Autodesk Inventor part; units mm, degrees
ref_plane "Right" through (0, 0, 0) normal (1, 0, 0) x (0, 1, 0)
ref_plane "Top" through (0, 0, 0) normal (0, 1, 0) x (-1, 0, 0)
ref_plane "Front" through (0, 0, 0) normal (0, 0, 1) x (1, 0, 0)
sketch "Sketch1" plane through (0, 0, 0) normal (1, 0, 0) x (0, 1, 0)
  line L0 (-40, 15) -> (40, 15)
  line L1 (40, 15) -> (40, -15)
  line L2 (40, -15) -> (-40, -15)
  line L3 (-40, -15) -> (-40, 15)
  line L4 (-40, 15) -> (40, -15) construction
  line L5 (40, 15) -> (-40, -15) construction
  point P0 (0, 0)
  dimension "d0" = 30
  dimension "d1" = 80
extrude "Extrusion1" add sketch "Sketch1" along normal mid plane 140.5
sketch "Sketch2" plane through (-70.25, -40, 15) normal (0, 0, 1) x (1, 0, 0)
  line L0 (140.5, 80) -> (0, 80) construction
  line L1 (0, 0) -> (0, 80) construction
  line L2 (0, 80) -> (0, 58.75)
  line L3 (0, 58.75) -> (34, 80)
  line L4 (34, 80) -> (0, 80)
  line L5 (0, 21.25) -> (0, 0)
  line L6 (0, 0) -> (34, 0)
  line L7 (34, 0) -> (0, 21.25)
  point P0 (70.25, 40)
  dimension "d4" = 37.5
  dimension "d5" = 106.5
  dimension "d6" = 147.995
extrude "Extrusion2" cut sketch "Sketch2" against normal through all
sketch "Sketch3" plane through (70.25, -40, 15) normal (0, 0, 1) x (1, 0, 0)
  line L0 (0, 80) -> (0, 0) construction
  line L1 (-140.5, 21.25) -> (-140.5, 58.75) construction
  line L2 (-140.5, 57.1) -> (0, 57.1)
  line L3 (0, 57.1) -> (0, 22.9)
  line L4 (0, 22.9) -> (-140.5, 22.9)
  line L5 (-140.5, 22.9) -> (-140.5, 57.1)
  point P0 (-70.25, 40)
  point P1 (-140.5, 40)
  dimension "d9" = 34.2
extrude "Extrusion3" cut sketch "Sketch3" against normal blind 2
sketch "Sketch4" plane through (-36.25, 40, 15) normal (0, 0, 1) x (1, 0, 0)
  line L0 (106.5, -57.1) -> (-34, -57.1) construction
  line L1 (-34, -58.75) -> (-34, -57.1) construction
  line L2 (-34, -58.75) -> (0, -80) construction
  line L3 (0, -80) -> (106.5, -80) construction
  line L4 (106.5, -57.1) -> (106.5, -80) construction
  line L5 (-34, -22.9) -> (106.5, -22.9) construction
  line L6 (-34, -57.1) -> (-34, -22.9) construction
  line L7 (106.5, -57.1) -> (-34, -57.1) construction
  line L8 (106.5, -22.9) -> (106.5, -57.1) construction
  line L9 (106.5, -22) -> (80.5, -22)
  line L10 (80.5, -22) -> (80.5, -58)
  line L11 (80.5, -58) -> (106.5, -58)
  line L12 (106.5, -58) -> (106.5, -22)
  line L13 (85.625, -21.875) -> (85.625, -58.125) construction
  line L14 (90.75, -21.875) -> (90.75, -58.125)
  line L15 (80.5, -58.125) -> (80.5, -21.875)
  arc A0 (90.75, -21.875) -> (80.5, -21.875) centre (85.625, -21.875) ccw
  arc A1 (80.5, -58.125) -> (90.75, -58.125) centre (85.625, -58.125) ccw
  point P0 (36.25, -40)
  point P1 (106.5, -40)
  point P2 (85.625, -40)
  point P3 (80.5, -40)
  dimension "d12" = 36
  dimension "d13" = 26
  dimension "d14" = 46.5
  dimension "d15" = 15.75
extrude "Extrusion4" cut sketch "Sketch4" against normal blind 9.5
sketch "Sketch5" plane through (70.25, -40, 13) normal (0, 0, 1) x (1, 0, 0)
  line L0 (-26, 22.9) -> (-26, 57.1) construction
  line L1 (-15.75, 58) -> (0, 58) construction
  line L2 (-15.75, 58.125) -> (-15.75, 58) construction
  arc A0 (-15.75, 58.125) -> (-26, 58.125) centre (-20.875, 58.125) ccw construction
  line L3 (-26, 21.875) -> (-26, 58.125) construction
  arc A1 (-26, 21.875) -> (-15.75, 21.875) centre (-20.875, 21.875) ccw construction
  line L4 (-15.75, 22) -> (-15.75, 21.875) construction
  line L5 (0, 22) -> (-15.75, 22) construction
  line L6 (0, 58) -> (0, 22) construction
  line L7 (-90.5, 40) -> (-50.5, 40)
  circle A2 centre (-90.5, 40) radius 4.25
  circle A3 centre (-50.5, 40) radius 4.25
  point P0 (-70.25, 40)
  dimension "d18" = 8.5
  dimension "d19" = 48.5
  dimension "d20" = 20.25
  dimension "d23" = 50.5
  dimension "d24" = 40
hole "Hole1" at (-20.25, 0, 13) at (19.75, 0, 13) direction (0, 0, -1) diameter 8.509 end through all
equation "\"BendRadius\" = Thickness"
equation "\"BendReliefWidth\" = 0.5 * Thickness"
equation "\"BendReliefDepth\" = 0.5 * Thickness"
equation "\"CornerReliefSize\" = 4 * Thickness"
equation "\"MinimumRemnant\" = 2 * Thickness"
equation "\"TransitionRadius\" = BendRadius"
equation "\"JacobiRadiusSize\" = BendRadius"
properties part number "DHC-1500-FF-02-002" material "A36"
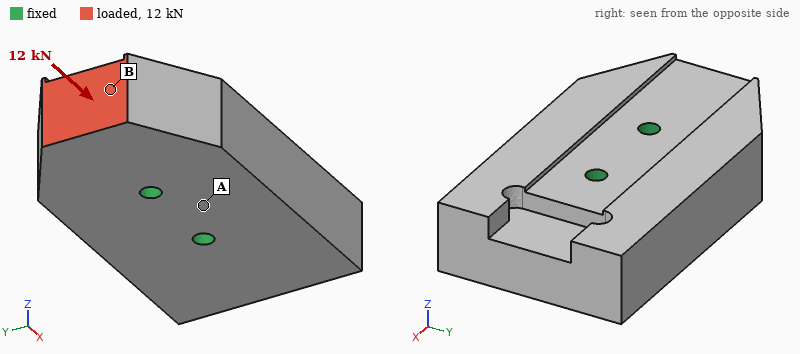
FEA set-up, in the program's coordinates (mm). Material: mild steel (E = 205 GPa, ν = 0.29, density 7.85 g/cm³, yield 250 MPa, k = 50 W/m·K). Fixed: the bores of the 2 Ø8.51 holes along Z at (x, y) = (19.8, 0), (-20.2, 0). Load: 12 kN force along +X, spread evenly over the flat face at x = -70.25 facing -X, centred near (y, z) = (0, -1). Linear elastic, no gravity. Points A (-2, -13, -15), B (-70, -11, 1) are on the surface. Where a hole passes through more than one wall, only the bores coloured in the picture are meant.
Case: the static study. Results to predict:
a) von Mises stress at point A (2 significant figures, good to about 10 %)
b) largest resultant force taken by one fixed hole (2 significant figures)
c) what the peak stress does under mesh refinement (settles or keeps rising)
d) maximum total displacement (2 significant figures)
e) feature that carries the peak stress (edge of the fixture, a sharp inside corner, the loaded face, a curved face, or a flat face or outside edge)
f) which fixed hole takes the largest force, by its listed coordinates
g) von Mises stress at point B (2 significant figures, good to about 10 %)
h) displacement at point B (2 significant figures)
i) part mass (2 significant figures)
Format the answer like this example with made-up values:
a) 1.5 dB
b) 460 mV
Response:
a) 3.0 MPa
b) 8.8 kN
c) keeps rising
d) 2.8 µm
e) edge of the fixture
f) (-20.2, 0)
g) 8.9 MPa
h) 2.4 µm
i) 2.3 kg
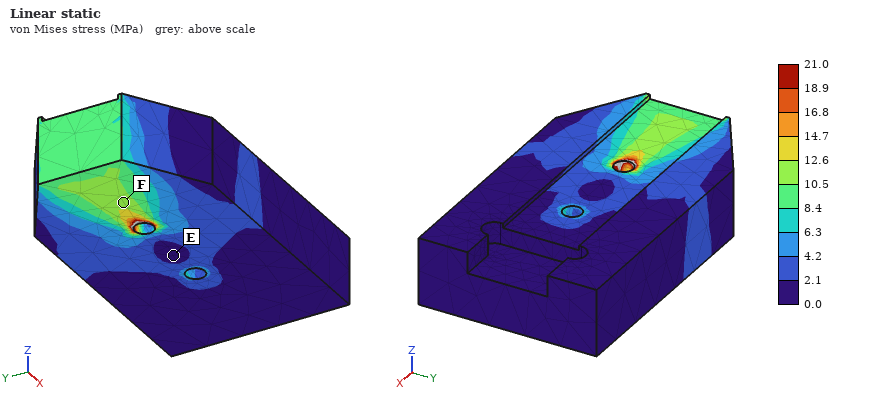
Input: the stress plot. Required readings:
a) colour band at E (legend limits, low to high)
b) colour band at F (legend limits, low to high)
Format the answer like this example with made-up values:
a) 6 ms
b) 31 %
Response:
a) 0.0 to 2.1 MPa
b) 10.5 to 12.6 MPa
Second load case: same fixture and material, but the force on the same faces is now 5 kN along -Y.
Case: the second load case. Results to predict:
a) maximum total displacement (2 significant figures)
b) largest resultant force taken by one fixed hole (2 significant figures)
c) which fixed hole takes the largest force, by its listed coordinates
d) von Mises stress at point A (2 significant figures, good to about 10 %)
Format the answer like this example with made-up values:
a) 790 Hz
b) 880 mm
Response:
a) 6.4 µm
b) 10 kN
c) (-20.2, 0)
d) 5.3 MPa
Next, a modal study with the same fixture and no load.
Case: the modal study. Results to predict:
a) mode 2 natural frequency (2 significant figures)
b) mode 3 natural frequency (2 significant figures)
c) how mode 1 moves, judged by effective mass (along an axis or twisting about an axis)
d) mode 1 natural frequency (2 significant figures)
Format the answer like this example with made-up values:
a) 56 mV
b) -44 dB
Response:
a) 6400 Hz
b) 6400 Hz
c) along Z
d) 5900 Hz
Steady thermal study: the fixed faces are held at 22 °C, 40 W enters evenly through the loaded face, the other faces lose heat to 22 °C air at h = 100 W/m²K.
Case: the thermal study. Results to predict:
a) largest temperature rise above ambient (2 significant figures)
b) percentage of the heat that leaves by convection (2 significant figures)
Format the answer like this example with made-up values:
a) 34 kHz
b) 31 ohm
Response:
a) 25 K
b) 30 %
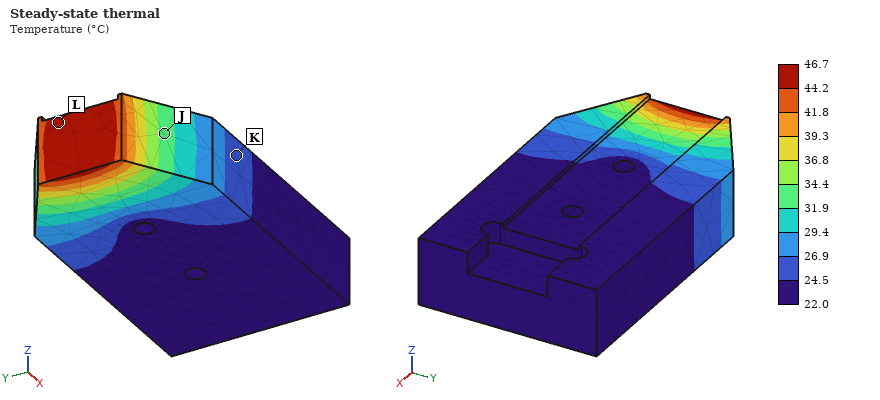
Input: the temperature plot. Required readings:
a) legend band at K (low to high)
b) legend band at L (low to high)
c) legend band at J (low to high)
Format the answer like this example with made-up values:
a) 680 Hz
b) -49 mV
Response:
a) 24.5 to 26.9 °C
b) 44.2 to 46.7 °C
c) 31.9 to 34.4 °C
